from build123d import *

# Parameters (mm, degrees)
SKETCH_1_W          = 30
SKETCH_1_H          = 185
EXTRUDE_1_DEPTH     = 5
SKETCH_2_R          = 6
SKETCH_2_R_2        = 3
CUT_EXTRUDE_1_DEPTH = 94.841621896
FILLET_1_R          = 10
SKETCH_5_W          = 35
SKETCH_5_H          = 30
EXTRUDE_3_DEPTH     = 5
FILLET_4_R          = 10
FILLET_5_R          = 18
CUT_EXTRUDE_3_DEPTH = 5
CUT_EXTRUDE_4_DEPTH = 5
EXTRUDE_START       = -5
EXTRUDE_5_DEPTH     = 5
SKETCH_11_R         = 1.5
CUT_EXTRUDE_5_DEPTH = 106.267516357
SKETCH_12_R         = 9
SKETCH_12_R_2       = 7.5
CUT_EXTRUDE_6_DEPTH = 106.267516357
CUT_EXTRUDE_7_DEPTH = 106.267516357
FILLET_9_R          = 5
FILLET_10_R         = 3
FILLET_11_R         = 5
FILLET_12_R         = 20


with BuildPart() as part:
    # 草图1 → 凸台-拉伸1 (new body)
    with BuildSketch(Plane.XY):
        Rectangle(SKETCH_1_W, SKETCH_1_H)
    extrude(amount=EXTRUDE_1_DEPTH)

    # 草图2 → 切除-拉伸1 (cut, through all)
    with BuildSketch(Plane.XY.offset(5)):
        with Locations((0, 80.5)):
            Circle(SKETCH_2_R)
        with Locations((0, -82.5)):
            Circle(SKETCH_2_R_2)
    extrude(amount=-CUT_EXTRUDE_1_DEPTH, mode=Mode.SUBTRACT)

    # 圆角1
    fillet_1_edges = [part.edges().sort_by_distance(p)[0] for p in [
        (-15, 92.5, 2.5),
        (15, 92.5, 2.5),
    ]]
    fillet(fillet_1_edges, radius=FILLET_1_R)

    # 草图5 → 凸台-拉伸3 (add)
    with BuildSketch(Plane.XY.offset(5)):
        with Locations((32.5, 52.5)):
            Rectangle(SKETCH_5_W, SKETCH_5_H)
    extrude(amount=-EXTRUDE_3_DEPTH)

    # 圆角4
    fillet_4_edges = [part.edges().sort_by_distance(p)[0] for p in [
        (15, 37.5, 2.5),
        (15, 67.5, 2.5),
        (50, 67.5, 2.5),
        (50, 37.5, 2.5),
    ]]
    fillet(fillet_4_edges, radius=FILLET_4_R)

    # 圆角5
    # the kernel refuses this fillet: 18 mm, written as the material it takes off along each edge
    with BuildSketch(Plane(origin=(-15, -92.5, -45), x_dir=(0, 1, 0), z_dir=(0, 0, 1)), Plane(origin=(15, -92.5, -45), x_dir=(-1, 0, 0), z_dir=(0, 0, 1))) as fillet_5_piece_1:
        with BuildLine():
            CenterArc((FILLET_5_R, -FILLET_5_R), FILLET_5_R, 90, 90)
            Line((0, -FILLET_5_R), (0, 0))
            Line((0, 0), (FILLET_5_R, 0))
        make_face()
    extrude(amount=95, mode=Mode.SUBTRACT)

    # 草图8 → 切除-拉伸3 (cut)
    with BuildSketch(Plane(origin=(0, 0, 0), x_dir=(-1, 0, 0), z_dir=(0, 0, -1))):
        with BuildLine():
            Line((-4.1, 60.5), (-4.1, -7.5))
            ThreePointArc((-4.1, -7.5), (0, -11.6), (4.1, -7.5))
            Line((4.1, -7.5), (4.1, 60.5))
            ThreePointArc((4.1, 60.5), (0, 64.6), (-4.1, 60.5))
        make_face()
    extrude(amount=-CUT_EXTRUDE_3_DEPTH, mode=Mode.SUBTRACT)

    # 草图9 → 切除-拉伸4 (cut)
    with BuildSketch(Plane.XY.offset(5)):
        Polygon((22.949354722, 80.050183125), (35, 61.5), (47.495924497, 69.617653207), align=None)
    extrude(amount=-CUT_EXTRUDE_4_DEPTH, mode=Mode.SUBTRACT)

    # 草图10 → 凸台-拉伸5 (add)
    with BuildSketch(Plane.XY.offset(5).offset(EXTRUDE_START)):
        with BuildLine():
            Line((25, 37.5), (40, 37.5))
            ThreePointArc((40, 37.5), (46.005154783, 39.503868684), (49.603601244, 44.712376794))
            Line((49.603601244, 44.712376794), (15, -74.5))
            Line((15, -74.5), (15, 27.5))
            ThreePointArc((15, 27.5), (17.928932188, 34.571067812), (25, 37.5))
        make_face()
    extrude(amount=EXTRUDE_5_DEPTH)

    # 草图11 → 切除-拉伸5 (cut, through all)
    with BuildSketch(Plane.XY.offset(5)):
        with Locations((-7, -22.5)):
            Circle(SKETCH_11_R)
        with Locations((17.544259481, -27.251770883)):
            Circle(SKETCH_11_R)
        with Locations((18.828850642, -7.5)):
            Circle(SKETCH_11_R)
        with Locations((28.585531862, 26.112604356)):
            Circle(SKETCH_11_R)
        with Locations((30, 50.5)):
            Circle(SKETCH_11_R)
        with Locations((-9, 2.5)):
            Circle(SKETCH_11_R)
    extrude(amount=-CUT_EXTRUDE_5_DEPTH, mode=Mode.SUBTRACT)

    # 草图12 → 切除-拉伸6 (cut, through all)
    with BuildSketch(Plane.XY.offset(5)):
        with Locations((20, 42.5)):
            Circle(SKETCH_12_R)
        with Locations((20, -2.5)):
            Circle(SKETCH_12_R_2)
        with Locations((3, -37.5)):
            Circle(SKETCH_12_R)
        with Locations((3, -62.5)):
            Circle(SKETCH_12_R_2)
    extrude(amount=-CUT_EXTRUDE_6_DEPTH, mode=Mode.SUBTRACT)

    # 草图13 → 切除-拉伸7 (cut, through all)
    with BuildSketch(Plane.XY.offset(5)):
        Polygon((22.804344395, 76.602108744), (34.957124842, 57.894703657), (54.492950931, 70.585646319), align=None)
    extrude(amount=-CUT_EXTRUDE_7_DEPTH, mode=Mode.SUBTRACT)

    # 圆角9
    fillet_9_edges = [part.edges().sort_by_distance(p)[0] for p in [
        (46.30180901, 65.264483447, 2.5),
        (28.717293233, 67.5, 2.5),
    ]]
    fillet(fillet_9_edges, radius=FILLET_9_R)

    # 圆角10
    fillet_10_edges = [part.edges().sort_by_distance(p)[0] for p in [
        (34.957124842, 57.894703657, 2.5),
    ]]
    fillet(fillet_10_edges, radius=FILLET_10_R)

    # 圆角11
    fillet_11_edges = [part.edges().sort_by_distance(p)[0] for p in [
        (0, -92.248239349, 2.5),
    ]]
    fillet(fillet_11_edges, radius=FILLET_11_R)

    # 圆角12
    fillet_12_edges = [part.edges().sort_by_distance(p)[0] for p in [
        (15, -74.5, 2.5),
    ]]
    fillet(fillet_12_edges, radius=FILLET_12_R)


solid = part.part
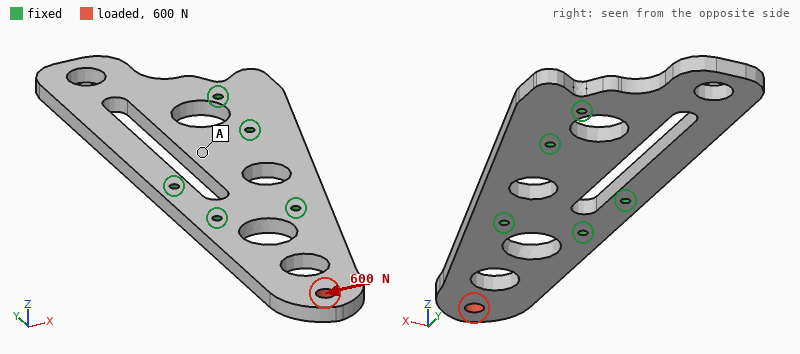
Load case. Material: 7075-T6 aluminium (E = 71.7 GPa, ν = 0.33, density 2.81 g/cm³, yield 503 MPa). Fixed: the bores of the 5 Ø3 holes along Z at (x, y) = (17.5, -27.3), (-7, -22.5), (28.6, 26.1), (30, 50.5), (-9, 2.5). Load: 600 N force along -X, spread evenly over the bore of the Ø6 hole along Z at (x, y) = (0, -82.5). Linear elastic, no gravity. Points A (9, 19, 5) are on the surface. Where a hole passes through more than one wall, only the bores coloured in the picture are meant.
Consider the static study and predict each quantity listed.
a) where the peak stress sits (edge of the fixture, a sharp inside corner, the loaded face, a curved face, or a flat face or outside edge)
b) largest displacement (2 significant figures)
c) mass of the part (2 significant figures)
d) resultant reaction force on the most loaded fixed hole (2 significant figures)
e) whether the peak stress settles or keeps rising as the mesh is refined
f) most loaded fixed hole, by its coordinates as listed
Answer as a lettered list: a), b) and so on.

a) edge of the fixture
b) 54 µm
c) 91 g
d) 1.1 kN
e) keeps rising
f) (17.5, -27.3)
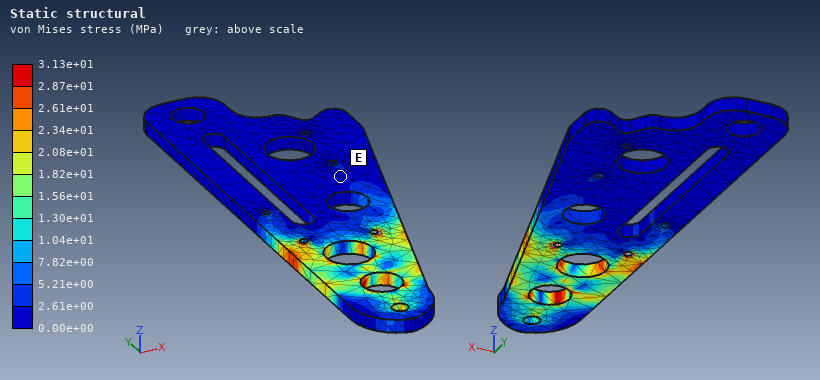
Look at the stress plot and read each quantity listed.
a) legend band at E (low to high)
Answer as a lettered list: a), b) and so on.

a) 0.00e+00 to 2.61e+00 MPa
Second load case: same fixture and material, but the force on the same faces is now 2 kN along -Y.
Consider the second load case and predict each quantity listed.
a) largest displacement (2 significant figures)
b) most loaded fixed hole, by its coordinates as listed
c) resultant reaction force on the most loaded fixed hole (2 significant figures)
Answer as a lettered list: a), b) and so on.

a) 26 µm
b) (-7, -22.5)
c) 1.2 kN
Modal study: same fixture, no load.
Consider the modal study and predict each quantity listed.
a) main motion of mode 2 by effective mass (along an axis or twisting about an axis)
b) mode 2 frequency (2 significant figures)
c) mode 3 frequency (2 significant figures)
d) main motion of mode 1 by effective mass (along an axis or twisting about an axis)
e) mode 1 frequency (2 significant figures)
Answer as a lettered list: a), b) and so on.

a) along Z
b) 1300 Hz
c) 3400 Hz
d) along Z
e) 970 Hz
